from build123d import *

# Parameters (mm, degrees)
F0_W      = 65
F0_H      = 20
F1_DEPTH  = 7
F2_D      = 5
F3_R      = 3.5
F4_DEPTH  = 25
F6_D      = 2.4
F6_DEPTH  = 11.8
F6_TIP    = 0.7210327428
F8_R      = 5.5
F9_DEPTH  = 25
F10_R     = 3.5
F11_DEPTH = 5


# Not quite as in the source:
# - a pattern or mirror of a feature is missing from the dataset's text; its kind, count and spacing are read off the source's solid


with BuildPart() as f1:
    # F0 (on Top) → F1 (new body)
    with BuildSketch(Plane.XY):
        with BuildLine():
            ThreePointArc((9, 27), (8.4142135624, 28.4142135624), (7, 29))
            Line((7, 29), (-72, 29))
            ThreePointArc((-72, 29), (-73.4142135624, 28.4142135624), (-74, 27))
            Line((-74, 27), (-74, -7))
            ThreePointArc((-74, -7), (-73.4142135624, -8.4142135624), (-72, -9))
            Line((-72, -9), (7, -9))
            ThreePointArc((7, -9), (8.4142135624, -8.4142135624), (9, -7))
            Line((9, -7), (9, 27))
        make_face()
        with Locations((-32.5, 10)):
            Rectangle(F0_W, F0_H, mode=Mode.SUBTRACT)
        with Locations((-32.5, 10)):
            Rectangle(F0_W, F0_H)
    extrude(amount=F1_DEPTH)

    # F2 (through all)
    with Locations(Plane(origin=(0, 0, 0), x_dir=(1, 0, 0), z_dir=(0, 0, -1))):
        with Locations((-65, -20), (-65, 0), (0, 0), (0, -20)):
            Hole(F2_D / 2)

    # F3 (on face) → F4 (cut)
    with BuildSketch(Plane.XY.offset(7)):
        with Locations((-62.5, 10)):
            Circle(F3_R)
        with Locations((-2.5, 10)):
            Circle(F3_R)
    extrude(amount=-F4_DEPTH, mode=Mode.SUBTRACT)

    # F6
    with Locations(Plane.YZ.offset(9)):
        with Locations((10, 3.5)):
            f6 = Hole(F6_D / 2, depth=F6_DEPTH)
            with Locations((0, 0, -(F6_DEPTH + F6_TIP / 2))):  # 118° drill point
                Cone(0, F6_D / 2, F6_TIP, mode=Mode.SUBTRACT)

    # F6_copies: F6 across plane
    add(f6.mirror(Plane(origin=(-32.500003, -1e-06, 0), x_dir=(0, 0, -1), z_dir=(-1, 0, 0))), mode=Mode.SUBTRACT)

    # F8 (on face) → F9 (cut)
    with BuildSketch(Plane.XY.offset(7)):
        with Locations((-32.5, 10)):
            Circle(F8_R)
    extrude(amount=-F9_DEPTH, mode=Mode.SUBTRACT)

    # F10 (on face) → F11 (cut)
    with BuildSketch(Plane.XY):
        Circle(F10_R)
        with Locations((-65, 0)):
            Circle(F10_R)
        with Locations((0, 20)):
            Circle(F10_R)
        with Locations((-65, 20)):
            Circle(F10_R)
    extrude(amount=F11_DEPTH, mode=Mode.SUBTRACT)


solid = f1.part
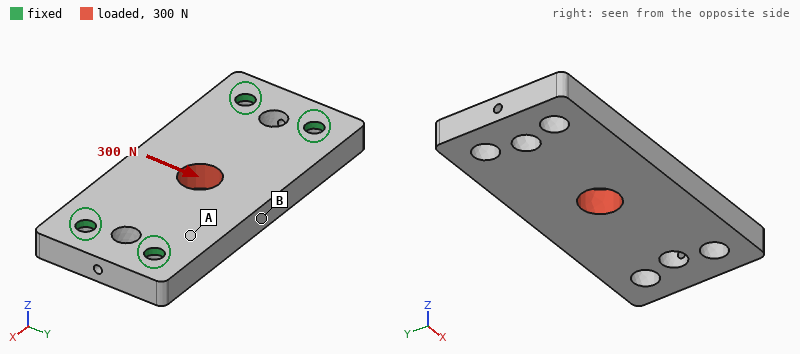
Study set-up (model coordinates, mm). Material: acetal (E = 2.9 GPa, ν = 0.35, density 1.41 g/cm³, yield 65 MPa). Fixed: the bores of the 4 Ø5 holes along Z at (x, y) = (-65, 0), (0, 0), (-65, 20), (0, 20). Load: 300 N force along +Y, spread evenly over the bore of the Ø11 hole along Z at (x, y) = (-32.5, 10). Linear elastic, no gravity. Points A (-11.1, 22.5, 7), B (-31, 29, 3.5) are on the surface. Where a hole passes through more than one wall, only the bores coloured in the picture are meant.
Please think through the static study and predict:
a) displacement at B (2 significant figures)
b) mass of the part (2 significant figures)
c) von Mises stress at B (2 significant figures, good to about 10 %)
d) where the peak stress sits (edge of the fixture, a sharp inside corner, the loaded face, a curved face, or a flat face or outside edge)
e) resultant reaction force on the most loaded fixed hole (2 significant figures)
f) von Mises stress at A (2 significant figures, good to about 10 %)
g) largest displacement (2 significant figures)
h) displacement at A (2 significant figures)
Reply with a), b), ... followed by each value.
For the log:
a) 31 µm
b) 28 g
c) 2.2 MPa
d) edge of the fixture
e) 97 N
f) 1.0 MPa
g) 35 µm
h) 16 µm
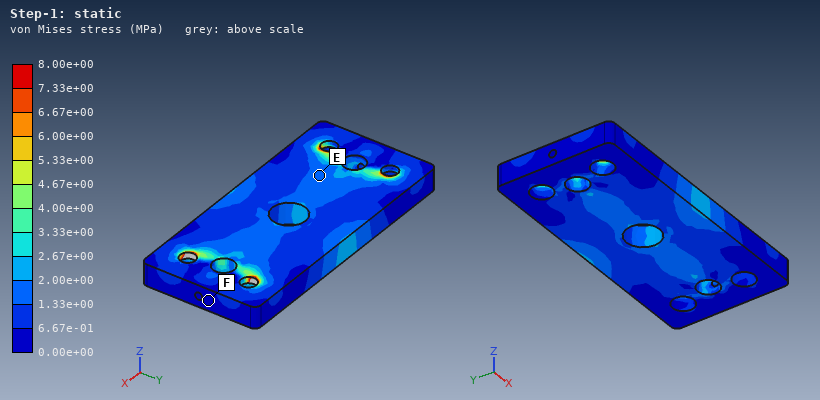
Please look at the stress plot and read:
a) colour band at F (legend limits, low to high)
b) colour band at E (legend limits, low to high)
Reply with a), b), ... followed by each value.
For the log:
a) 0.00e+00 to 6.67e-01 MPa
b) 1.33e+00 to 2.00e+00 MPa
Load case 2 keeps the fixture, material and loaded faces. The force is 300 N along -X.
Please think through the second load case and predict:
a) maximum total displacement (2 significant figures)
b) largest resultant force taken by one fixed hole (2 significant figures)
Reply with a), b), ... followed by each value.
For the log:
a) 14 µm
b) 76 N
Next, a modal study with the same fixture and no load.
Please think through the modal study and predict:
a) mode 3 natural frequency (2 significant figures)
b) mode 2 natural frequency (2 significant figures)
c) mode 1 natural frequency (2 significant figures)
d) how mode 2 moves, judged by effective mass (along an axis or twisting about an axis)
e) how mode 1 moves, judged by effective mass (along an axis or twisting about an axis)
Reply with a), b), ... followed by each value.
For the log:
a) 4100 Hz
b) 2600 Hz
c) 1700 Hz
d) twisting about X
e) along Z
